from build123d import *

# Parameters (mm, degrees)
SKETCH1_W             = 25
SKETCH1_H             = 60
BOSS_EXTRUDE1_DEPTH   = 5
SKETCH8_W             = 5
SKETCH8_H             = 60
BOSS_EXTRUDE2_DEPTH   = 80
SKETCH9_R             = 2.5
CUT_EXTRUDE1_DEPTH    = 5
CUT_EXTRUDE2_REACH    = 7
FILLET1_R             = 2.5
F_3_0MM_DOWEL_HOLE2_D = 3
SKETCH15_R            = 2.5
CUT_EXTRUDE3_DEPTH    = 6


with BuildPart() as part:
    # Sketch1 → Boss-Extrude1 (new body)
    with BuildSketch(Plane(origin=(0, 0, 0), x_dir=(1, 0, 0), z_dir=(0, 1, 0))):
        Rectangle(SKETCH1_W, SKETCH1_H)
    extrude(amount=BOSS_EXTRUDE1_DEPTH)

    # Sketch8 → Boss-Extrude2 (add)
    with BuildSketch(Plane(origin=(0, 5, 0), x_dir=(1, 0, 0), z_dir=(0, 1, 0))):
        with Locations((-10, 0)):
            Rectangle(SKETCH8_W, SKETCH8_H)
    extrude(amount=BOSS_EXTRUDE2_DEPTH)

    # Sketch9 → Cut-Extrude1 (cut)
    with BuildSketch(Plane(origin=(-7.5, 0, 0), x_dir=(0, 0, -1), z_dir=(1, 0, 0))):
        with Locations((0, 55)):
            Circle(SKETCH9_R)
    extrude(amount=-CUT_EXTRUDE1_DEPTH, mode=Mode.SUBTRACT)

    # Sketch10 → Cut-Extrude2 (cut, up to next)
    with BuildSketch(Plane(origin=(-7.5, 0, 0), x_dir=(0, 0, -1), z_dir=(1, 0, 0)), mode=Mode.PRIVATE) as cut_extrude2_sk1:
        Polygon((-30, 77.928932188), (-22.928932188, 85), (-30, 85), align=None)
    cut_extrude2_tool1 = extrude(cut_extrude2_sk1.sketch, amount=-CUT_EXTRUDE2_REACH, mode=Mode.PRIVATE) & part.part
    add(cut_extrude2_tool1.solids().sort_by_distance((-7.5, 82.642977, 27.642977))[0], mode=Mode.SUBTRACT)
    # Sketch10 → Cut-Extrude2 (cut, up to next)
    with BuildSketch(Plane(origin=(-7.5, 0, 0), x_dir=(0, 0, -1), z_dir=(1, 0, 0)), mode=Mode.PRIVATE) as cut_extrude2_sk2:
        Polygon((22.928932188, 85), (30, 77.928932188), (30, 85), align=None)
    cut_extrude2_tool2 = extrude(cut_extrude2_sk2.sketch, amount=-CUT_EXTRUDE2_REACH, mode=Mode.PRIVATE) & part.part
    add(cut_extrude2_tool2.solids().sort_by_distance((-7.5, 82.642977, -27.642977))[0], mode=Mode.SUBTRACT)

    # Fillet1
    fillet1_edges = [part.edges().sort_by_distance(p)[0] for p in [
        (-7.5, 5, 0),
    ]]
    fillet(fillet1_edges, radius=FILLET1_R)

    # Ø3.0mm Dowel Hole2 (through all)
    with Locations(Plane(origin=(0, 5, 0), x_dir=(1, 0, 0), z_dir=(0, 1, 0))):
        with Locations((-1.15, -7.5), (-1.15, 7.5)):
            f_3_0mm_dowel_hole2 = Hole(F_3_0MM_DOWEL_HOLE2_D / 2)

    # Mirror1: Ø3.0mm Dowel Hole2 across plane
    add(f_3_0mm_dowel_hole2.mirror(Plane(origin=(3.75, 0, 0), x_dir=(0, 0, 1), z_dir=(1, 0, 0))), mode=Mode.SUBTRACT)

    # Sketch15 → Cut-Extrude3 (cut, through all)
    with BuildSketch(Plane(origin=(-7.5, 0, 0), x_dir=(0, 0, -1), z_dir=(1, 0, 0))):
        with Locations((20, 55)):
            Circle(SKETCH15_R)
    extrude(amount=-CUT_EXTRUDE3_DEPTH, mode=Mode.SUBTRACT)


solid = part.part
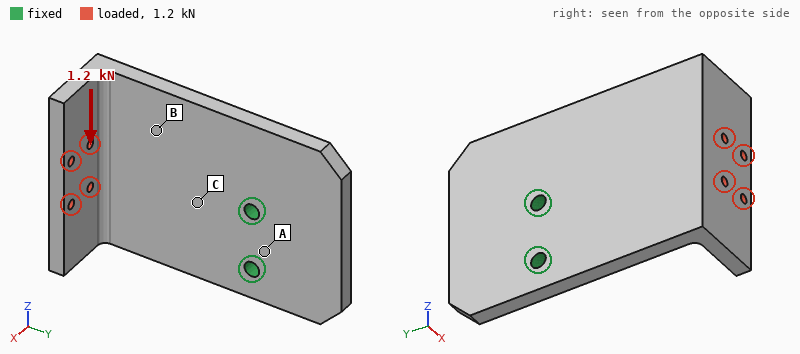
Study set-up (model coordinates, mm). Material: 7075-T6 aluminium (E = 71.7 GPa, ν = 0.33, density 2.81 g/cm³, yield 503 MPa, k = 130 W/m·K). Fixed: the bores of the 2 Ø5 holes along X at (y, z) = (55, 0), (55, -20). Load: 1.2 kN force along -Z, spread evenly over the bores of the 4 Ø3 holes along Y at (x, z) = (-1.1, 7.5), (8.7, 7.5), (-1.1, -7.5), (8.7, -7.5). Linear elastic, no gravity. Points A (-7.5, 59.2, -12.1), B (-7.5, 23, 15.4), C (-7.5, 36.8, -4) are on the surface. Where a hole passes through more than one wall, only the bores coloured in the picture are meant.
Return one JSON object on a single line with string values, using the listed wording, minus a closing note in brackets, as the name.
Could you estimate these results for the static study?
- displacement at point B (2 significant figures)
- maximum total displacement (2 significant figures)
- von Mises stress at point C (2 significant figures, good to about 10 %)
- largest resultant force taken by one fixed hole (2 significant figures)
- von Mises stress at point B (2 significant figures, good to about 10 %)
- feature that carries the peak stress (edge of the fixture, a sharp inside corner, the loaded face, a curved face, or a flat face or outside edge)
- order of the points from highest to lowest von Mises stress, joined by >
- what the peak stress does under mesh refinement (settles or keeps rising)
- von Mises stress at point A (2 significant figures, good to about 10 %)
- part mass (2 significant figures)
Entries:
{"displacement at point B": "0.14 mm", "maximum total displacement": "0.43 mm", "von Mises stress at point C": "67 MPa", "largest resultant force taken by one fixed hole": "2.8 kN", "von Mises stress at point B": "45 MPa", "feature that carries the peak stress": "edge of the fixture", "order of the points from highest to lowest von Mises stress, joined by >": "C > B > A", "what the peak stress does under mesh refinement": "keeps rising", "von Mises stress at point A": "17 MPa", "part mass": "87 g"}
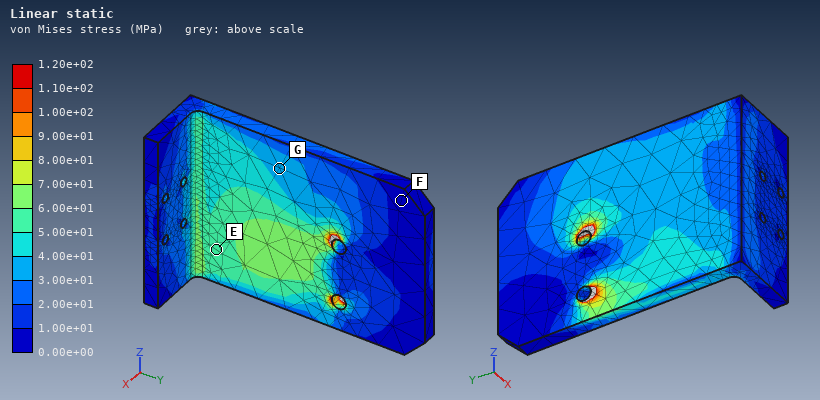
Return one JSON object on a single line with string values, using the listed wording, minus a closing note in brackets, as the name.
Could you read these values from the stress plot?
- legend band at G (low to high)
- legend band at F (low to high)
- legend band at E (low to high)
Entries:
{"legend band at G": "3.00e+01 to 4.00e+01 MPa", "legend band at F": "0.00e+00 to 1.00e+01 MPa", "legend band at E": "5.00e+01 to 6.00e+01 MPa"}
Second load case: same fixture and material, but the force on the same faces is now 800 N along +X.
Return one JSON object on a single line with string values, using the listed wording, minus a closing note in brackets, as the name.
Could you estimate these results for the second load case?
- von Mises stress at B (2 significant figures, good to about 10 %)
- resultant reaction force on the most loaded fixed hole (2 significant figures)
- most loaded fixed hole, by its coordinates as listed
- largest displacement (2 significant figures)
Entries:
{"von Mises stress at B": "57 MPa", "resultant reaction force on the most loaded fixed hole": "650 N", "most loaded fixed hole, by its coordinates as listed": "(55, 0)", "largest displacement": "1.2 mm"}
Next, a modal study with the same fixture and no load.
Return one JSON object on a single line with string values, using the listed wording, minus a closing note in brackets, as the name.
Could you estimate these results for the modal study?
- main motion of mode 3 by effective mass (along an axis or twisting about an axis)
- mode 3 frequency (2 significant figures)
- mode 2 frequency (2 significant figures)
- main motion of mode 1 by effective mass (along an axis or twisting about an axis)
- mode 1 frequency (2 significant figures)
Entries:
{"main motion of mode 3 by effective mass": "along X", "mode 3 frequency": "3700 Hz", "mode 2 frequency": "1700 Hz", "main motion of mode 1 by effective mass": "along X", "mode 1 frequency": "820 Hz"}
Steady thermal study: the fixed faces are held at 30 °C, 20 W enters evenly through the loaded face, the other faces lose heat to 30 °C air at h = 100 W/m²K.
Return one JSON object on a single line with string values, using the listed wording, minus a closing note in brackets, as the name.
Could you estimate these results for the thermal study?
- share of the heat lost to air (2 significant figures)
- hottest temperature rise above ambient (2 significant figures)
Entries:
{"share of the heat lost to air": "57 %", "hottest temperature rise above ambient": "24 K"}
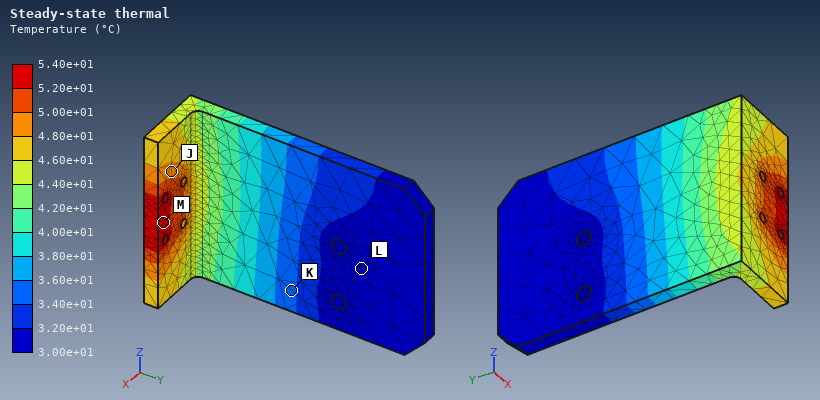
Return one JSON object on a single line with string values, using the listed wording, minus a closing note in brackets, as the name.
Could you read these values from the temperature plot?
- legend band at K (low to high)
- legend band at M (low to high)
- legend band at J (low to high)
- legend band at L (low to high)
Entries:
{"legend band at K": "3.40e+01 to 3.60e+01 °C", "legend band at M": "5.20e+01 to 5.40e+01 °C", "legend band at J": "4.80e+01 to 5.00e+01 °C", "legend band at L": "3.00e+01 to 3.20e+01 °C"}
